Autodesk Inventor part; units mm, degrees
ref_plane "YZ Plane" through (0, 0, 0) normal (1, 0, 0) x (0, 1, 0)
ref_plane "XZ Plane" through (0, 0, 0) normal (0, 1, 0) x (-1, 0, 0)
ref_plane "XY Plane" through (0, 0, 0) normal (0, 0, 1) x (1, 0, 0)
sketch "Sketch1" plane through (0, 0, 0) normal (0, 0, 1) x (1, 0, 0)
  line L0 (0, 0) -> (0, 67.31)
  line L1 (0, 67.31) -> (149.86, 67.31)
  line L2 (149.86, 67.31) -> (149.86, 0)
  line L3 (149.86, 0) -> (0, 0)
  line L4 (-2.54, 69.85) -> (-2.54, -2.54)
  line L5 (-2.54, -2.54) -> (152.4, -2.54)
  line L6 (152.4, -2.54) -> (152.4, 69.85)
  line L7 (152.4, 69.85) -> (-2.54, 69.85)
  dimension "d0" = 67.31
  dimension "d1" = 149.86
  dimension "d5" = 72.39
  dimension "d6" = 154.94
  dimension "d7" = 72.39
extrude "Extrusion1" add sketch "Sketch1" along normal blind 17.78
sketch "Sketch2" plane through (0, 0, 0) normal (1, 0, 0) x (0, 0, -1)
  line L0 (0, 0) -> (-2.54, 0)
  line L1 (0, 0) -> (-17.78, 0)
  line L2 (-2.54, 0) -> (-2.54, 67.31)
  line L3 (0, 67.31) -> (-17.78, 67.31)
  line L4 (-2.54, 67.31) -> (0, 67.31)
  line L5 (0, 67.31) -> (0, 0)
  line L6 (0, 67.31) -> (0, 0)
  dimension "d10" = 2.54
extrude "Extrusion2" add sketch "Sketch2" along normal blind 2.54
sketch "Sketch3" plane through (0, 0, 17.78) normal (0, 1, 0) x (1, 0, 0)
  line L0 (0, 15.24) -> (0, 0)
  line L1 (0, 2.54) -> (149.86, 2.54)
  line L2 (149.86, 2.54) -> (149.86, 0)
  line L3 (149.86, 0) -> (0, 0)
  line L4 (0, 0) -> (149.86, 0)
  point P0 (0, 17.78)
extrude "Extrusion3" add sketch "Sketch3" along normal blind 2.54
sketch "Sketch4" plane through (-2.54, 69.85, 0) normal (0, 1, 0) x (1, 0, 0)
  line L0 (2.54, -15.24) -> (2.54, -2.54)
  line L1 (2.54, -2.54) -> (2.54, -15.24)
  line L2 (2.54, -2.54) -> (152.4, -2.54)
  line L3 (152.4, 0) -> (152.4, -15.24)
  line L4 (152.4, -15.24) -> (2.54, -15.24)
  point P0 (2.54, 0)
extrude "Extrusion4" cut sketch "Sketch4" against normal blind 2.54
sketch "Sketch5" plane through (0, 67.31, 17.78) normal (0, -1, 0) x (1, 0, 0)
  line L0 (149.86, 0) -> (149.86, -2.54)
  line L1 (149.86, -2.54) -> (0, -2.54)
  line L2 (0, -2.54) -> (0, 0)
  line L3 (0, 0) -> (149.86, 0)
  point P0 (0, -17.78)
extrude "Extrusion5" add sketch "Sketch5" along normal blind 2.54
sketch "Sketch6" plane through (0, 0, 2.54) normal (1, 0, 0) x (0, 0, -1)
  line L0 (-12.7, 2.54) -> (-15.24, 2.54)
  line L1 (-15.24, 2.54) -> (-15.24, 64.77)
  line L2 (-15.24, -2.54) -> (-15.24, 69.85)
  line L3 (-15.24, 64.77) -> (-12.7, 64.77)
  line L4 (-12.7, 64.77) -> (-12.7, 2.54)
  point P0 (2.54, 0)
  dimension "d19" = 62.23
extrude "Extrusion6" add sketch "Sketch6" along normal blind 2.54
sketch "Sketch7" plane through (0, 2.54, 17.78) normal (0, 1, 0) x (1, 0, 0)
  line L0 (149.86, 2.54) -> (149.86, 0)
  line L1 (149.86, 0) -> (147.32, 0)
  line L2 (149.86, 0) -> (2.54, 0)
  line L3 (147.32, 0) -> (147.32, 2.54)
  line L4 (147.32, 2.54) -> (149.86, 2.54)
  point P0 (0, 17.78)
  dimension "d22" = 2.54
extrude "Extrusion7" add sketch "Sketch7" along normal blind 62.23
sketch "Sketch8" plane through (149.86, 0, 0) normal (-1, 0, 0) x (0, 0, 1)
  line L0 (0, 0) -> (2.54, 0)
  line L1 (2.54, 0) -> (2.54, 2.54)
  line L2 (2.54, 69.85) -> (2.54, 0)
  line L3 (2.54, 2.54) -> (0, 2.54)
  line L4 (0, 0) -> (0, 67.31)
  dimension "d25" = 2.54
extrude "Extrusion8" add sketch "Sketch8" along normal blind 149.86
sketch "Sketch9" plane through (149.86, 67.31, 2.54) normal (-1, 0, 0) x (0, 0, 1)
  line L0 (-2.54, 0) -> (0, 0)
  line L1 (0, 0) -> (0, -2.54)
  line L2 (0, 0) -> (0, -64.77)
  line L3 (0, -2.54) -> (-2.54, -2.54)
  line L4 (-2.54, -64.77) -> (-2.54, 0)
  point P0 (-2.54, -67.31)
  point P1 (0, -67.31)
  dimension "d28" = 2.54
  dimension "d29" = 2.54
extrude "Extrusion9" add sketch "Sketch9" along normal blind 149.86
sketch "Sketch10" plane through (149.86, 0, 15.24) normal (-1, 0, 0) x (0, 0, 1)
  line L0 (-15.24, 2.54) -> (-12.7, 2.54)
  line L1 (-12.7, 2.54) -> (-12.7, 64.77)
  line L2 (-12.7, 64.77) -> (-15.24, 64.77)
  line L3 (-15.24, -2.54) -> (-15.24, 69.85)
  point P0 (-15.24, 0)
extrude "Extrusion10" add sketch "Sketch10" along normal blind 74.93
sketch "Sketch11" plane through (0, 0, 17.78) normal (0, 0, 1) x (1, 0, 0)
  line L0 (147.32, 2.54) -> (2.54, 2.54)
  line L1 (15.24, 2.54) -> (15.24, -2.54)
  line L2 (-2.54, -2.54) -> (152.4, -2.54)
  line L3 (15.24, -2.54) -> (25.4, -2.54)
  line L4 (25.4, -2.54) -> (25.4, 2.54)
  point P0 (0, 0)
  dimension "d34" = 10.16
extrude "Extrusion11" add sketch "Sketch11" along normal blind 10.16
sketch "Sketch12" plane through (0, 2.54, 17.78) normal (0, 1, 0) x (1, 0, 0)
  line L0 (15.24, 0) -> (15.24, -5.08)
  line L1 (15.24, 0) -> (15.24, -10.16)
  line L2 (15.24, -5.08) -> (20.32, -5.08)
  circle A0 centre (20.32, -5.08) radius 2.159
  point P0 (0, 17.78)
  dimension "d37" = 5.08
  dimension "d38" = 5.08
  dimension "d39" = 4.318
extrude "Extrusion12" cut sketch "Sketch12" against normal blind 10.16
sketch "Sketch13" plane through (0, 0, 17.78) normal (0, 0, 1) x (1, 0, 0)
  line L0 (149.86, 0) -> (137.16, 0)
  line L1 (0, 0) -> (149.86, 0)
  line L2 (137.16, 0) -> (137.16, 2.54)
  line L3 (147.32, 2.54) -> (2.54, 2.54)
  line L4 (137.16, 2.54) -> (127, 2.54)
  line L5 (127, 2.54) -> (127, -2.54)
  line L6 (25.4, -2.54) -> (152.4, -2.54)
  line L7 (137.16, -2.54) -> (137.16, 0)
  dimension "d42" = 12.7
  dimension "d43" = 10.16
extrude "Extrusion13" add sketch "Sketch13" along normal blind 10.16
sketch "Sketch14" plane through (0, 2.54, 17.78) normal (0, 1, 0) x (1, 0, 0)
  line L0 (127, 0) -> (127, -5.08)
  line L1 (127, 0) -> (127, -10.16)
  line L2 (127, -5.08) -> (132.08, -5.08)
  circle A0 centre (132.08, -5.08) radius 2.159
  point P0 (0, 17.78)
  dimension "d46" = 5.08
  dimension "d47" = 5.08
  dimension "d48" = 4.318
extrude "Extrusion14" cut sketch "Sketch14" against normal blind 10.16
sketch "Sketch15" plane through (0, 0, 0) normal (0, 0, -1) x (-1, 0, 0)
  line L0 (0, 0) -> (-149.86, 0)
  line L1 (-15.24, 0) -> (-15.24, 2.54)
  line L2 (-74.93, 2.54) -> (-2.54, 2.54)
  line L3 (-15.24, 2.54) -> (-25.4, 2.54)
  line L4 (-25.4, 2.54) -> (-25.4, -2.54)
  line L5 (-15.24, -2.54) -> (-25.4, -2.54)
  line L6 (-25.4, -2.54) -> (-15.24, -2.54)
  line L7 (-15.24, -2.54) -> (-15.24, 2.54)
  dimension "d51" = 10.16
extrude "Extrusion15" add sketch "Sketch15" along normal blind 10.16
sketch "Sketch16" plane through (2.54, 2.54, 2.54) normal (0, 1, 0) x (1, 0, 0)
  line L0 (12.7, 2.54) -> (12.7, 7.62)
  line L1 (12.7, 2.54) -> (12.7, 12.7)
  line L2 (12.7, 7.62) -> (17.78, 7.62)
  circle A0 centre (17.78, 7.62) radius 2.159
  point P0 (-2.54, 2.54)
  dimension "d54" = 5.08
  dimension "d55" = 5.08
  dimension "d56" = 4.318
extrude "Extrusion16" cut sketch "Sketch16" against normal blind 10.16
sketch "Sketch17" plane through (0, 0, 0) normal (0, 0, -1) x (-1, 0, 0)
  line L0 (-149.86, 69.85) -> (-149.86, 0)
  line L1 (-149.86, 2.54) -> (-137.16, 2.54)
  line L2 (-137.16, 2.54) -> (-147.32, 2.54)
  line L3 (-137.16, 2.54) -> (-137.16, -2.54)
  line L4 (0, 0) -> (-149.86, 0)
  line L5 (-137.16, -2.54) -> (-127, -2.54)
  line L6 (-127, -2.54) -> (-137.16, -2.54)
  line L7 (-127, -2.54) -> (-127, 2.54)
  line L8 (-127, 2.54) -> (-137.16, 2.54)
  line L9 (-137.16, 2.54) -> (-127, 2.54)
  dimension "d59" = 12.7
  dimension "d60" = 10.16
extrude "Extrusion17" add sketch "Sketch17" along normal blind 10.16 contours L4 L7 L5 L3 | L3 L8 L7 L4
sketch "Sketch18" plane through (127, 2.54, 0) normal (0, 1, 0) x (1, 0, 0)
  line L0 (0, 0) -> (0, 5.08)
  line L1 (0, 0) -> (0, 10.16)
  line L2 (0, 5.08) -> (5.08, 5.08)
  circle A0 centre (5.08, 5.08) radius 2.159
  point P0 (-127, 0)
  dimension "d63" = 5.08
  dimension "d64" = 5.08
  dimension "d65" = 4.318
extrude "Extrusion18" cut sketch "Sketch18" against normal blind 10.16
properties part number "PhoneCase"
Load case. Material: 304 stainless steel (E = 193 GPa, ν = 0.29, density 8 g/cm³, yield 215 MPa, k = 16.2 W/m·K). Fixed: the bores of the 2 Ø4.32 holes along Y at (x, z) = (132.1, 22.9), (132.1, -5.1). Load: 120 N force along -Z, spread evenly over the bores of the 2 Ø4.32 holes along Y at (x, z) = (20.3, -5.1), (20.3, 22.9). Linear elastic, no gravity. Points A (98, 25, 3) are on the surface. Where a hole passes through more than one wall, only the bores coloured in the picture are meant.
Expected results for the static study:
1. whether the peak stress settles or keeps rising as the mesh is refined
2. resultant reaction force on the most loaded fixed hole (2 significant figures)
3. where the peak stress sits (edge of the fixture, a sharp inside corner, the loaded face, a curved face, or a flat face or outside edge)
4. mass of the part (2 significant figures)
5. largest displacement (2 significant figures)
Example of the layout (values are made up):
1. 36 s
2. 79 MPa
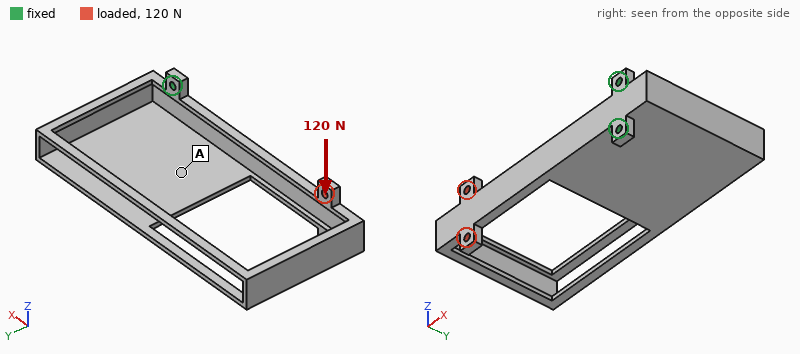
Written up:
1. keeps rising
2. 600 N
3. a sharp inside corner
4. 270 g
5. 0.20 mm
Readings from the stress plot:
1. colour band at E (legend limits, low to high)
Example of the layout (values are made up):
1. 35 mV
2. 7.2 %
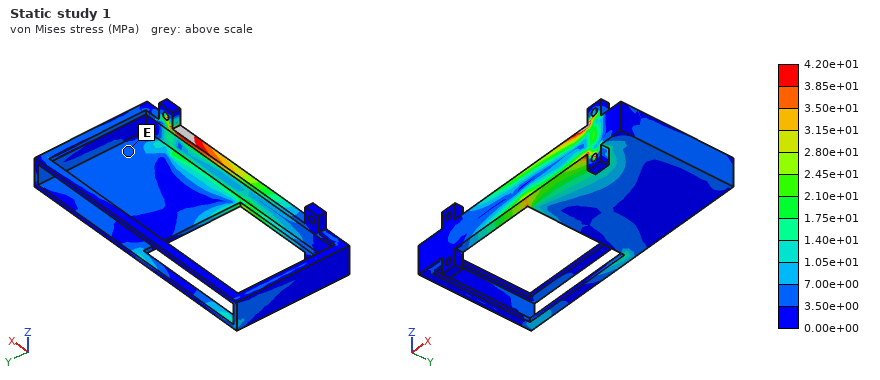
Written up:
1. 3.50e+00 to 7.00e+00 MPa
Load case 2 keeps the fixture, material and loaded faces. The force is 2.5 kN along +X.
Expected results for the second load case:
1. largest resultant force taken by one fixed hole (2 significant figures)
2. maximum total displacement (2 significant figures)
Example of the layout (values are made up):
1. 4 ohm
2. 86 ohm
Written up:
1. 1.3 kN
2. 69 µm
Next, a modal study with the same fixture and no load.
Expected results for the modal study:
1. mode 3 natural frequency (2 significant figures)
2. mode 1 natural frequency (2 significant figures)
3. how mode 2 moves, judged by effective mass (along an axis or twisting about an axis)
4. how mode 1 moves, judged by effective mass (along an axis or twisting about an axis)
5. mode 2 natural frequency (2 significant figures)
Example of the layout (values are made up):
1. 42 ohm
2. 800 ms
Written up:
1. 560 Hz
2. 200 Hz
3. along Y
4. along Z
5. 260 Hz
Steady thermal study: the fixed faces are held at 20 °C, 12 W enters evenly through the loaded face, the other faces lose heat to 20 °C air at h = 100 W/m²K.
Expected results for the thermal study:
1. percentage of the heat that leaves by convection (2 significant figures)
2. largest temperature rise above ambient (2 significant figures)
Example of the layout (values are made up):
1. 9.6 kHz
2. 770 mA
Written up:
1. 100 %
2. 87 K
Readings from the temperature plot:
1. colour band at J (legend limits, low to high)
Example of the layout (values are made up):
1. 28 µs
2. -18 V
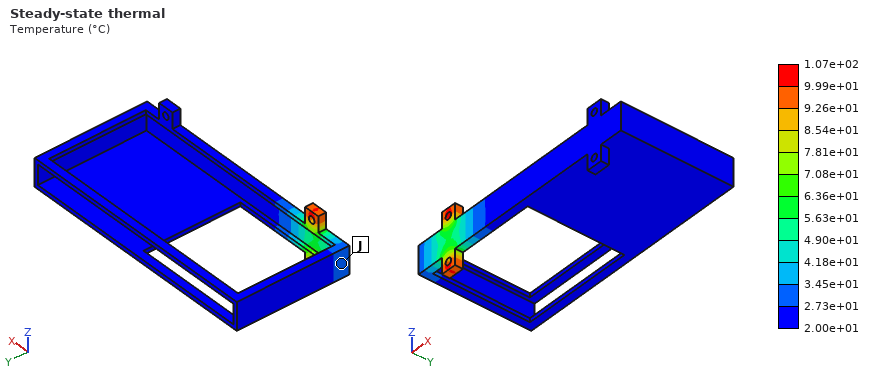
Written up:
1. 2.73e+01 to 3.45e+01 °C
